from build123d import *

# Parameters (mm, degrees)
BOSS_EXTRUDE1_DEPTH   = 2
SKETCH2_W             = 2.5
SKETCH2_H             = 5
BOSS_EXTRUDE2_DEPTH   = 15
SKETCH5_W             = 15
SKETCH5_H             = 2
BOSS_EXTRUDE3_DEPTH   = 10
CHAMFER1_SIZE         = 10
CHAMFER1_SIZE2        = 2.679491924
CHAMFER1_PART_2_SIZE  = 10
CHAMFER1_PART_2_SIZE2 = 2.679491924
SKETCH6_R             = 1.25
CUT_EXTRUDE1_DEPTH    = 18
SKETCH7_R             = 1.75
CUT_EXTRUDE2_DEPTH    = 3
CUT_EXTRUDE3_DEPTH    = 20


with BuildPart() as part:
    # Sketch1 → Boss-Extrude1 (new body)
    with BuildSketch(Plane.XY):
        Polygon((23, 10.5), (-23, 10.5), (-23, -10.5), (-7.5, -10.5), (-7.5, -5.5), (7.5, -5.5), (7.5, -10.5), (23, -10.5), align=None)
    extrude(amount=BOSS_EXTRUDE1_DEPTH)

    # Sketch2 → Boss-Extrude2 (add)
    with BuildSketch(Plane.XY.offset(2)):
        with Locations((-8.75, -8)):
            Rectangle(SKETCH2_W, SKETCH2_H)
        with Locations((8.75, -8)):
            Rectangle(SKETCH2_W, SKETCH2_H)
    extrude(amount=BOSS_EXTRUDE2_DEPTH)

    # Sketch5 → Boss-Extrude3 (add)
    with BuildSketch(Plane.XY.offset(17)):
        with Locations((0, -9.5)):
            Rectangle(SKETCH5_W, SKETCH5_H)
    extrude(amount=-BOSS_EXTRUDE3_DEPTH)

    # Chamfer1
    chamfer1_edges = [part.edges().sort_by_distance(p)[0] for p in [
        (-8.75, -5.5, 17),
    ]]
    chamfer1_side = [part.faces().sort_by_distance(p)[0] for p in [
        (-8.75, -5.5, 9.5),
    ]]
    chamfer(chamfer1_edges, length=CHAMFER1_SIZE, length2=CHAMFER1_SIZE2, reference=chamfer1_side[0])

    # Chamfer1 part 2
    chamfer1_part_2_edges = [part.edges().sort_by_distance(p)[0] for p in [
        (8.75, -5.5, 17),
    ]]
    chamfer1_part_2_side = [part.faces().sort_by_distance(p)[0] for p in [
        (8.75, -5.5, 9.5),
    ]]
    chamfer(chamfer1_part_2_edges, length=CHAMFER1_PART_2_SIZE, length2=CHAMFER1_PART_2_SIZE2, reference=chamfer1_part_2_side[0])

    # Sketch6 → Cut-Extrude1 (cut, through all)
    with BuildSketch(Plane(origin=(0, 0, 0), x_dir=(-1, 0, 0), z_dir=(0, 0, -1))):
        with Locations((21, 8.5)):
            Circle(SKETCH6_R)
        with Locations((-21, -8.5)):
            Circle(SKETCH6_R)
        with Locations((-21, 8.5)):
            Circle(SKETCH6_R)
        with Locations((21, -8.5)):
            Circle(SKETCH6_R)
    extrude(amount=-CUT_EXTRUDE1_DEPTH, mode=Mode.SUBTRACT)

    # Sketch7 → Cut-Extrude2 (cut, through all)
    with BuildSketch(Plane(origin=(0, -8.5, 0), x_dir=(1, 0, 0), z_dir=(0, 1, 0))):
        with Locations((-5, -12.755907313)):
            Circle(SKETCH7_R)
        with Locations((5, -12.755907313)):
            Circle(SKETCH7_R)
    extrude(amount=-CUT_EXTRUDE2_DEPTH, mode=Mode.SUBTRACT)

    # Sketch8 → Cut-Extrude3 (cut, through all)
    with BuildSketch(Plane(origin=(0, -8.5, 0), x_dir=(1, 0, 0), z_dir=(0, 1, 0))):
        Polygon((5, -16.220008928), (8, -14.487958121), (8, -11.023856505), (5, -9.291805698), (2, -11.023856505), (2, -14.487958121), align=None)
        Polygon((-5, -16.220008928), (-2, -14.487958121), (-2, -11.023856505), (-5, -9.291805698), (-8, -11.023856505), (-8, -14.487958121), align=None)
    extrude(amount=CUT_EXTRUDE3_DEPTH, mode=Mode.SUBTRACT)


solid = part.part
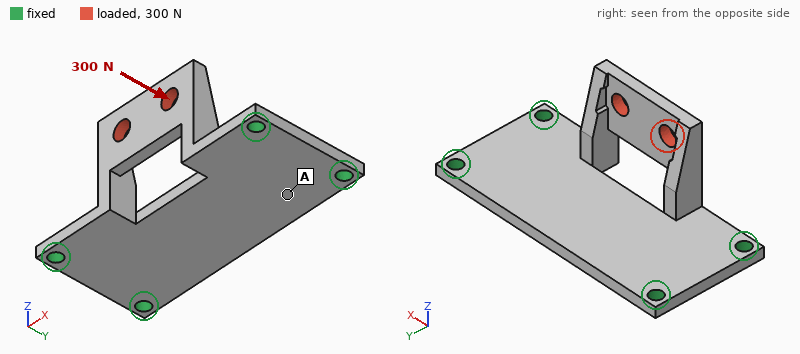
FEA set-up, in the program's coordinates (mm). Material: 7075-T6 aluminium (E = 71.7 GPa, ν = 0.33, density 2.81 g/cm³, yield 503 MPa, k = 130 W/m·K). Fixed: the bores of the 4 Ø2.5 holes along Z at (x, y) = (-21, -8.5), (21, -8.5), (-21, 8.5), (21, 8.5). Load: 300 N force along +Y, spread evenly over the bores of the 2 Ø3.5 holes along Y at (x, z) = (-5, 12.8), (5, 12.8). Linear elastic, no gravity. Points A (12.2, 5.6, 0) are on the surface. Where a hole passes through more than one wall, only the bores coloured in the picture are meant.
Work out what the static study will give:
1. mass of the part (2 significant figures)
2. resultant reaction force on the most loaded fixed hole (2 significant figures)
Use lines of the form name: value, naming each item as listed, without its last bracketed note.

mass of the part: 6.5 g
resultant reaction force on the most loaded fixed hole: 190 N
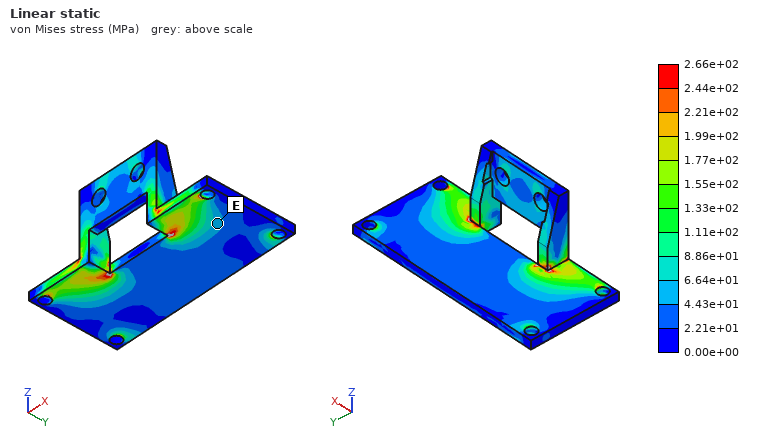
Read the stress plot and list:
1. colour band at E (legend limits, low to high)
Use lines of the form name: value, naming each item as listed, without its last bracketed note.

colour band at E: 4.43e+01 to 6.64e+01 MPa
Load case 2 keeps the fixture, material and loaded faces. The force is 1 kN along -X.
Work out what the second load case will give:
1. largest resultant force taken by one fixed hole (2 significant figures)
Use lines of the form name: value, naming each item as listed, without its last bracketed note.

largest resultant force taken by one fixed hole: 500 N
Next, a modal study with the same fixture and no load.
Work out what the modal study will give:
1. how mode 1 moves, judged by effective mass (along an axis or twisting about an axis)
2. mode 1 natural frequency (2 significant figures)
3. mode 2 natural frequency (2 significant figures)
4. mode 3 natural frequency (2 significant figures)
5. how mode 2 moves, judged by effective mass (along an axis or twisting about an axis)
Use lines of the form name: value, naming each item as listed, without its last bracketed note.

how mode 1 moves, judged by effective mass: along Y
mode 1 natural frequency: 4600 Hz
mode 2 natural frequency: 5900 Hz
mode 3 natural frequency: 8800 Hz
how mode 2 moves, judged by effective mass: along Z
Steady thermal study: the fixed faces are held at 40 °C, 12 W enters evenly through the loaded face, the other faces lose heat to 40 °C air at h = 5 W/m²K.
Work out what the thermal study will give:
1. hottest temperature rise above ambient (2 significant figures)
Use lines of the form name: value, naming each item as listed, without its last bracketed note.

hottest temperature rise above ambient: 69 K
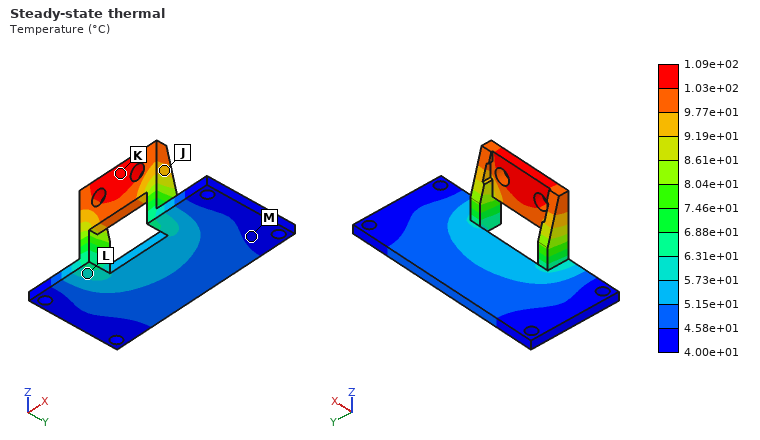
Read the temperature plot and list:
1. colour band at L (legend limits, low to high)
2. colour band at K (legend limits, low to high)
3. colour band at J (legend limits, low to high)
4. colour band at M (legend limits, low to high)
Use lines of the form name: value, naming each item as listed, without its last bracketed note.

colour band at L: 5.73e+01 to 6.31e+01 °C
colour band at K: 1.03e+02 to 1.09e+02 °C
colour band at J: 9.19e+01 to 9.77e+01 °C
colour band at M: 4.00e+01 to 4.58e+01 °C
